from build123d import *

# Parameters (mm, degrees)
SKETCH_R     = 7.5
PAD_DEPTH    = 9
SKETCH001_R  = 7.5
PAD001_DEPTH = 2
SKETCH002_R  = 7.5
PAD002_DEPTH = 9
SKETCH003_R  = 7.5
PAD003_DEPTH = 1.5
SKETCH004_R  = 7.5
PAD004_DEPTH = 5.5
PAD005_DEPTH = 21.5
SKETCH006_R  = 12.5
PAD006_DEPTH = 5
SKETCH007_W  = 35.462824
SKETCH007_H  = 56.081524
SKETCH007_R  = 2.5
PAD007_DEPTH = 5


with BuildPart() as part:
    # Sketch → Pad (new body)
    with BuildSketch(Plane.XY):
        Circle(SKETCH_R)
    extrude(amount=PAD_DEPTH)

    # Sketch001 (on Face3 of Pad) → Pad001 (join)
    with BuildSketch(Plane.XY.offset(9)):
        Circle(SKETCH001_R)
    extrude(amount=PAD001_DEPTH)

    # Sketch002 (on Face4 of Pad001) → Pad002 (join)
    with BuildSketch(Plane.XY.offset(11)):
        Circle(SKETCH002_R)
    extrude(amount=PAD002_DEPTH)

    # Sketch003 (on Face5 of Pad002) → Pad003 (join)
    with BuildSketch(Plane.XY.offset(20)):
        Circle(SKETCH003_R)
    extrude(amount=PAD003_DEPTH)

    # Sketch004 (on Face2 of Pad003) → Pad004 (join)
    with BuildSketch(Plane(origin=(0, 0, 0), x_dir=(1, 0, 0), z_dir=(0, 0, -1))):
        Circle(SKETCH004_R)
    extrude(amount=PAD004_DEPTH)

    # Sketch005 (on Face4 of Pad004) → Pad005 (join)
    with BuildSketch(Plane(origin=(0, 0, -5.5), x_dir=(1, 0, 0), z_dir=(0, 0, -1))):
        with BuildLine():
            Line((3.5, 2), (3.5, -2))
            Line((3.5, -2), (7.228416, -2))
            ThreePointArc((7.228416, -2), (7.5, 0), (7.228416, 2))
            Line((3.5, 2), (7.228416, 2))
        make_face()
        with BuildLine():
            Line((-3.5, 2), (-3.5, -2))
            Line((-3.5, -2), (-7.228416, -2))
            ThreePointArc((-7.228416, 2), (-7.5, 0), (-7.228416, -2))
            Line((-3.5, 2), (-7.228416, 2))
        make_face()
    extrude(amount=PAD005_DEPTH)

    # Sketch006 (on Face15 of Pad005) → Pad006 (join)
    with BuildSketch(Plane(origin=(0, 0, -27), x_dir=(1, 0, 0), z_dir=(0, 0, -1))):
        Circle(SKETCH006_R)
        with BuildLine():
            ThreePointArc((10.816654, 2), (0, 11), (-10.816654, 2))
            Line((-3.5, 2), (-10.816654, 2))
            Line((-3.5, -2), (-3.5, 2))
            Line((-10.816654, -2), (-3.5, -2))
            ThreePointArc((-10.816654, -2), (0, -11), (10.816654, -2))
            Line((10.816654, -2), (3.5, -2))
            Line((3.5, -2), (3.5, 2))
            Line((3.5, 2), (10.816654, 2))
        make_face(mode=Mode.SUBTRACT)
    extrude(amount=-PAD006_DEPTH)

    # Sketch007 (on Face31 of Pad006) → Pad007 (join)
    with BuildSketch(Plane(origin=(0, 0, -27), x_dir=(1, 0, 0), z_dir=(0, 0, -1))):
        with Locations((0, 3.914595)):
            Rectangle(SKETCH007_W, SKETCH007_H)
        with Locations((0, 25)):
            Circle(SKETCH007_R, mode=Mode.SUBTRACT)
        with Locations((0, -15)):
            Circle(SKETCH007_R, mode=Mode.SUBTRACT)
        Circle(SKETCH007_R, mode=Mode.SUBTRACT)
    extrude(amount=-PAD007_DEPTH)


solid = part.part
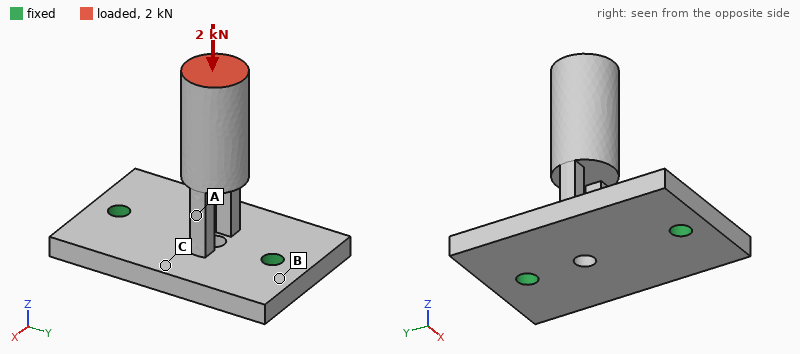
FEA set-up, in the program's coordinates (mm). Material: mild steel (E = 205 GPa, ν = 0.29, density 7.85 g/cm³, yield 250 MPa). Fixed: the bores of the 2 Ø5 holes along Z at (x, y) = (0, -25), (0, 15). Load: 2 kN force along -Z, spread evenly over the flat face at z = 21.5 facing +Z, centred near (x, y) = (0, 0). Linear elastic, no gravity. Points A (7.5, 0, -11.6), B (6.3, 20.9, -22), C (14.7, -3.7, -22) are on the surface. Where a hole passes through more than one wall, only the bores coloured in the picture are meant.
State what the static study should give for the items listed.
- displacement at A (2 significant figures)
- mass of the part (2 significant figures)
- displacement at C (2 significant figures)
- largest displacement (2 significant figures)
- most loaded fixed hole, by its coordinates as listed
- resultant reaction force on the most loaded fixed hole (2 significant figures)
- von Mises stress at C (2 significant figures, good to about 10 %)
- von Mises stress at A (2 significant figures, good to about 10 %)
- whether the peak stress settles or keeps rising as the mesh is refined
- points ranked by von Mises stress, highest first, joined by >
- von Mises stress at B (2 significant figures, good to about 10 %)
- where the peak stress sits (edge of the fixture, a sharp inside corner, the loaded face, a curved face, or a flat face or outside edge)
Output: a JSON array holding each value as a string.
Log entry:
["16 µm", "120 g", "12 µm", "27 µm", "(0, 15)", "1.3 kN", "39 MPa", "56 MPa", "keeps rising", "A > C > B", "16 MPa", "edge of the fixture"]
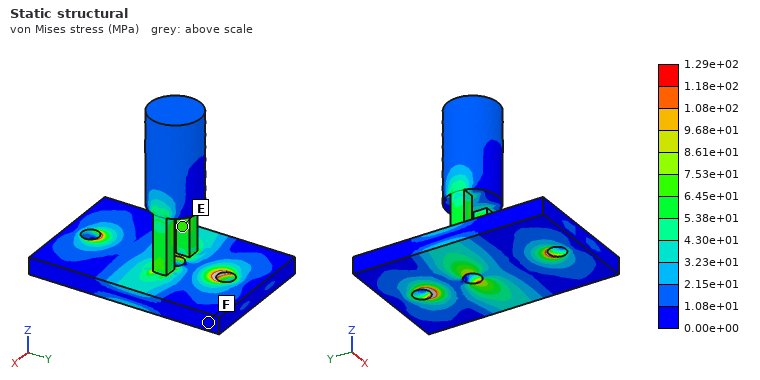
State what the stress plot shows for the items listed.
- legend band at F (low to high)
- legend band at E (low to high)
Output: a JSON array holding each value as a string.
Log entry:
["0.00e+00 to 1.08e+01 MPa", "6.45e+01 to 7.53e+01 MPa"]
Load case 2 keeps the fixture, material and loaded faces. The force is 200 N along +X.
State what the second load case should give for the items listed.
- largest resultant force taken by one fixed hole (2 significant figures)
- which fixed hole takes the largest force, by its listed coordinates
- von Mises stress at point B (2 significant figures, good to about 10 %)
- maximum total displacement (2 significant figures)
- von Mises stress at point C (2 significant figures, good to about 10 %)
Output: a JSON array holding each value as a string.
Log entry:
["130 N", "(0, 15)", "18 MPa", "74 µm", "17 MPa"]
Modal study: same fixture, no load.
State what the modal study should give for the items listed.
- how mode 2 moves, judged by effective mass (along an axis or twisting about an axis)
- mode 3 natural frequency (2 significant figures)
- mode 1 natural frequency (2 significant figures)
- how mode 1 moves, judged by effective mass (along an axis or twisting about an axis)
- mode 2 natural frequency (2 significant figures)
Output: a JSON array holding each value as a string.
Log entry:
["along X", "4100 Hz", "710 Hz", "along Y", "1800 Hz"]
